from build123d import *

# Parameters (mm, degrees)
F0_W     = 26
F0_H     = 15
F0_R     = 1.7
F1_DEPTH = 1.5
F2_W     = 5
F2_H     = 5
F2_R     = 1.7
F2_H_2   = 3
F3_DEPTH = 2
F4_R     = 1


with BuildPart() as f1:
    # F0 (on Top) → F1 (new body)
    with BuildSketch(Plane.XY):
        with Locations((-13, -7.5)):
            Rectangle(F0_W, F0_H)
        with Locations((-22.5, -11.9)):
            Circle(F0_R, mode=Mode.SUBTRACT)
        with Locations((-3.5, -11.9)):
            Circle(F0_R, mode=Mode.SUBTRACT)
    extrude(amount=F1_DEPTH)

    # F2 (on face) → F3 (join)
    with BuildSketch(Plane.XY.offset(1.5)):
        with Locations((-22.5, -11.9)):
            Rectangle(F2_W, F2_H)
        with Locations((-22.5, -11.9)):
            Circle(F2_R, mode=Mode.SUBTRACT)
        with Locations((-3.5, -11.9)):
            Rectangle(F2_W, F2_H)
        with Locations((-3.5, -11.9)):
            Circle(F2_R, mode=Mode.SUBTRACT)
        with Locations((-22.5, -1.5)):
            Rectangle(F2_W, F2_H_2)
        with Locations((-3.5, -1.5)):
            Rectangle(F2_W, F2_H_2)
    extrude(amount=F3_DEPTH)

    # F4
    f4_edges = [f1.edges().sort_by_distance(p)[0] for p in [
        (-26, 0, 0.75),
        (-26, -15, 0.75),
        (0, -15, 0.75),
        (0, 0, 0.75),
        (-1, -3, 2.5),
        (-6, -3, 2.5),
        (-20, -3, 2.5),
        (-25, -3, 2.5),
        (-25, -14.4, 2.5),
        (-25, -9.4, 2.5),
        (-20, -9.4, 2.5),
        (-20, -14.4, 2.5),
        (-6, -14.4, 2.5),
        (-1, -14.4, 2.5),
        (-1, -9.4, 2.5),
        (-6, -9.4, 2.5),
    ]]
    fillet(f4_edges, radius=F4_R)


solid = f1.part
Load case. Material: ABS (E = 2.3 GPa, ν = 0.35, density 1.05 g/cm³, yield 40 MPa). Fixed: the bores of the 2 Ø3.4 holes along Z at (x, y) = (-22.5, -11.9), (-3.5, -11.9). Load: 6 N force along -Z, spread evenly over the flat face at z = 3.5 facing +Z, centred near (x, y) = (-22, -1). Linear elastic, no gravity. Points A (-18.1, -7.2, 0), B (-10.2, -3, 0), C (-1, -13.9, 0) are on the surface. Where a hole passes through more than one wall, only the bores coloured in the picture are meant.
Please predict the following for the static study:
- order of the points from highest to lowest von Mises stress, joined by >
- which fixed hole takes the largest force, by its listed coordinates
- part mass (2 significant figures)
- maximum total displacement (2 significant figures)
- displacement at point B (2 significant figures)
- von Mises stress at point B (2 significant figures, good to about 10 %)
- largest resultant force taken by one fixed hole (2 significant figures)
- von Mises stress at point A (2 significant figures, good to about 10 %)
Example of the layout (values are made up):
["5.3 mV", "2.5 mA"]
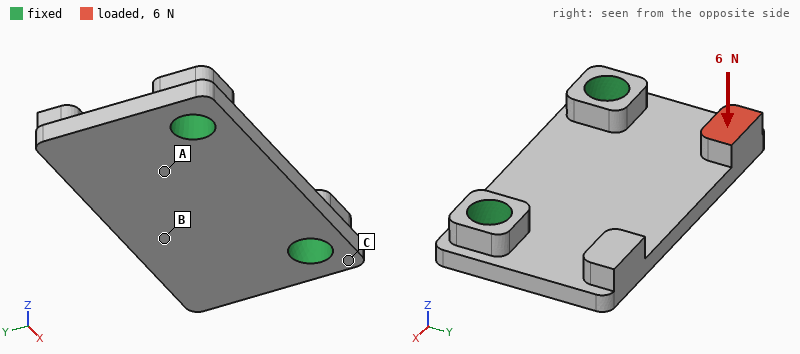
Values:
["A > B > C", "(-22.5, -11.9)", "0.71 g", "0.23 mm", "0.054 mm", "2.1 MPa", "6.0 N", "4.7 MPa"]
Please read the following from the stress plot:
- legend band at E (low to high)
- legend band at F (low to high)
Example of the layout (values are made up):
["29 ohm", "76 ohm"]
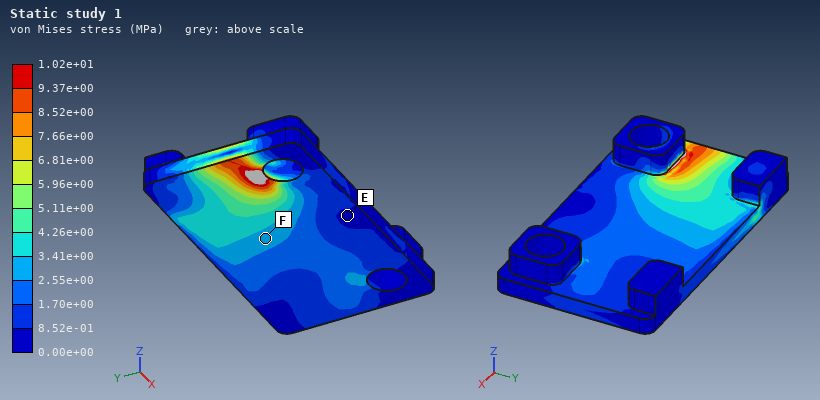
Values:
["0.00e+00 to 8.52e-01 MPa", "2.55e+00 to 3.41e+00 MPa"]
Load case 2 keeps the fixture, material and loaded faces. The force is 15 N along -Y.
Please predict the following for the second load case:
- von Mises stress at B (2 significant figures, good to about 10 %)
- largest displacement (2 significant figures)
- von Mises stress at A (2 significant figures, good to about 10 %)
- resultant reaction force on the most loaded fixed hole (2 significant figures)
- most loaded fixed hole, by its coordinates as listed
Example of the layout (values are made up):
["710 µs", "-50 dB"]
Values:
["2.8 MPa", "0.27 mm", "4.9 MPa", "15 N", "(-22.5, -11.9)"]
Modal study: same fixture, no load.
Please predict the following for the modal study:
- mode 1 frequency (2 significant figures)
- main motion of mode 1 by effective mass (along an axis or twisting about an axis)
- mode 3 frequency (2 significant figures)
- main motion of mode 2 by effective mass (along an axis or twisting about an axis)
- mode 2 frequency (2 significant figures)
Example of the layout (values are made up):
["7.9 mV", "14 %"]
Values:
["2500 Hz", "along Z", "5900 Hz", "twisting about Y", "3700 Hz"]
